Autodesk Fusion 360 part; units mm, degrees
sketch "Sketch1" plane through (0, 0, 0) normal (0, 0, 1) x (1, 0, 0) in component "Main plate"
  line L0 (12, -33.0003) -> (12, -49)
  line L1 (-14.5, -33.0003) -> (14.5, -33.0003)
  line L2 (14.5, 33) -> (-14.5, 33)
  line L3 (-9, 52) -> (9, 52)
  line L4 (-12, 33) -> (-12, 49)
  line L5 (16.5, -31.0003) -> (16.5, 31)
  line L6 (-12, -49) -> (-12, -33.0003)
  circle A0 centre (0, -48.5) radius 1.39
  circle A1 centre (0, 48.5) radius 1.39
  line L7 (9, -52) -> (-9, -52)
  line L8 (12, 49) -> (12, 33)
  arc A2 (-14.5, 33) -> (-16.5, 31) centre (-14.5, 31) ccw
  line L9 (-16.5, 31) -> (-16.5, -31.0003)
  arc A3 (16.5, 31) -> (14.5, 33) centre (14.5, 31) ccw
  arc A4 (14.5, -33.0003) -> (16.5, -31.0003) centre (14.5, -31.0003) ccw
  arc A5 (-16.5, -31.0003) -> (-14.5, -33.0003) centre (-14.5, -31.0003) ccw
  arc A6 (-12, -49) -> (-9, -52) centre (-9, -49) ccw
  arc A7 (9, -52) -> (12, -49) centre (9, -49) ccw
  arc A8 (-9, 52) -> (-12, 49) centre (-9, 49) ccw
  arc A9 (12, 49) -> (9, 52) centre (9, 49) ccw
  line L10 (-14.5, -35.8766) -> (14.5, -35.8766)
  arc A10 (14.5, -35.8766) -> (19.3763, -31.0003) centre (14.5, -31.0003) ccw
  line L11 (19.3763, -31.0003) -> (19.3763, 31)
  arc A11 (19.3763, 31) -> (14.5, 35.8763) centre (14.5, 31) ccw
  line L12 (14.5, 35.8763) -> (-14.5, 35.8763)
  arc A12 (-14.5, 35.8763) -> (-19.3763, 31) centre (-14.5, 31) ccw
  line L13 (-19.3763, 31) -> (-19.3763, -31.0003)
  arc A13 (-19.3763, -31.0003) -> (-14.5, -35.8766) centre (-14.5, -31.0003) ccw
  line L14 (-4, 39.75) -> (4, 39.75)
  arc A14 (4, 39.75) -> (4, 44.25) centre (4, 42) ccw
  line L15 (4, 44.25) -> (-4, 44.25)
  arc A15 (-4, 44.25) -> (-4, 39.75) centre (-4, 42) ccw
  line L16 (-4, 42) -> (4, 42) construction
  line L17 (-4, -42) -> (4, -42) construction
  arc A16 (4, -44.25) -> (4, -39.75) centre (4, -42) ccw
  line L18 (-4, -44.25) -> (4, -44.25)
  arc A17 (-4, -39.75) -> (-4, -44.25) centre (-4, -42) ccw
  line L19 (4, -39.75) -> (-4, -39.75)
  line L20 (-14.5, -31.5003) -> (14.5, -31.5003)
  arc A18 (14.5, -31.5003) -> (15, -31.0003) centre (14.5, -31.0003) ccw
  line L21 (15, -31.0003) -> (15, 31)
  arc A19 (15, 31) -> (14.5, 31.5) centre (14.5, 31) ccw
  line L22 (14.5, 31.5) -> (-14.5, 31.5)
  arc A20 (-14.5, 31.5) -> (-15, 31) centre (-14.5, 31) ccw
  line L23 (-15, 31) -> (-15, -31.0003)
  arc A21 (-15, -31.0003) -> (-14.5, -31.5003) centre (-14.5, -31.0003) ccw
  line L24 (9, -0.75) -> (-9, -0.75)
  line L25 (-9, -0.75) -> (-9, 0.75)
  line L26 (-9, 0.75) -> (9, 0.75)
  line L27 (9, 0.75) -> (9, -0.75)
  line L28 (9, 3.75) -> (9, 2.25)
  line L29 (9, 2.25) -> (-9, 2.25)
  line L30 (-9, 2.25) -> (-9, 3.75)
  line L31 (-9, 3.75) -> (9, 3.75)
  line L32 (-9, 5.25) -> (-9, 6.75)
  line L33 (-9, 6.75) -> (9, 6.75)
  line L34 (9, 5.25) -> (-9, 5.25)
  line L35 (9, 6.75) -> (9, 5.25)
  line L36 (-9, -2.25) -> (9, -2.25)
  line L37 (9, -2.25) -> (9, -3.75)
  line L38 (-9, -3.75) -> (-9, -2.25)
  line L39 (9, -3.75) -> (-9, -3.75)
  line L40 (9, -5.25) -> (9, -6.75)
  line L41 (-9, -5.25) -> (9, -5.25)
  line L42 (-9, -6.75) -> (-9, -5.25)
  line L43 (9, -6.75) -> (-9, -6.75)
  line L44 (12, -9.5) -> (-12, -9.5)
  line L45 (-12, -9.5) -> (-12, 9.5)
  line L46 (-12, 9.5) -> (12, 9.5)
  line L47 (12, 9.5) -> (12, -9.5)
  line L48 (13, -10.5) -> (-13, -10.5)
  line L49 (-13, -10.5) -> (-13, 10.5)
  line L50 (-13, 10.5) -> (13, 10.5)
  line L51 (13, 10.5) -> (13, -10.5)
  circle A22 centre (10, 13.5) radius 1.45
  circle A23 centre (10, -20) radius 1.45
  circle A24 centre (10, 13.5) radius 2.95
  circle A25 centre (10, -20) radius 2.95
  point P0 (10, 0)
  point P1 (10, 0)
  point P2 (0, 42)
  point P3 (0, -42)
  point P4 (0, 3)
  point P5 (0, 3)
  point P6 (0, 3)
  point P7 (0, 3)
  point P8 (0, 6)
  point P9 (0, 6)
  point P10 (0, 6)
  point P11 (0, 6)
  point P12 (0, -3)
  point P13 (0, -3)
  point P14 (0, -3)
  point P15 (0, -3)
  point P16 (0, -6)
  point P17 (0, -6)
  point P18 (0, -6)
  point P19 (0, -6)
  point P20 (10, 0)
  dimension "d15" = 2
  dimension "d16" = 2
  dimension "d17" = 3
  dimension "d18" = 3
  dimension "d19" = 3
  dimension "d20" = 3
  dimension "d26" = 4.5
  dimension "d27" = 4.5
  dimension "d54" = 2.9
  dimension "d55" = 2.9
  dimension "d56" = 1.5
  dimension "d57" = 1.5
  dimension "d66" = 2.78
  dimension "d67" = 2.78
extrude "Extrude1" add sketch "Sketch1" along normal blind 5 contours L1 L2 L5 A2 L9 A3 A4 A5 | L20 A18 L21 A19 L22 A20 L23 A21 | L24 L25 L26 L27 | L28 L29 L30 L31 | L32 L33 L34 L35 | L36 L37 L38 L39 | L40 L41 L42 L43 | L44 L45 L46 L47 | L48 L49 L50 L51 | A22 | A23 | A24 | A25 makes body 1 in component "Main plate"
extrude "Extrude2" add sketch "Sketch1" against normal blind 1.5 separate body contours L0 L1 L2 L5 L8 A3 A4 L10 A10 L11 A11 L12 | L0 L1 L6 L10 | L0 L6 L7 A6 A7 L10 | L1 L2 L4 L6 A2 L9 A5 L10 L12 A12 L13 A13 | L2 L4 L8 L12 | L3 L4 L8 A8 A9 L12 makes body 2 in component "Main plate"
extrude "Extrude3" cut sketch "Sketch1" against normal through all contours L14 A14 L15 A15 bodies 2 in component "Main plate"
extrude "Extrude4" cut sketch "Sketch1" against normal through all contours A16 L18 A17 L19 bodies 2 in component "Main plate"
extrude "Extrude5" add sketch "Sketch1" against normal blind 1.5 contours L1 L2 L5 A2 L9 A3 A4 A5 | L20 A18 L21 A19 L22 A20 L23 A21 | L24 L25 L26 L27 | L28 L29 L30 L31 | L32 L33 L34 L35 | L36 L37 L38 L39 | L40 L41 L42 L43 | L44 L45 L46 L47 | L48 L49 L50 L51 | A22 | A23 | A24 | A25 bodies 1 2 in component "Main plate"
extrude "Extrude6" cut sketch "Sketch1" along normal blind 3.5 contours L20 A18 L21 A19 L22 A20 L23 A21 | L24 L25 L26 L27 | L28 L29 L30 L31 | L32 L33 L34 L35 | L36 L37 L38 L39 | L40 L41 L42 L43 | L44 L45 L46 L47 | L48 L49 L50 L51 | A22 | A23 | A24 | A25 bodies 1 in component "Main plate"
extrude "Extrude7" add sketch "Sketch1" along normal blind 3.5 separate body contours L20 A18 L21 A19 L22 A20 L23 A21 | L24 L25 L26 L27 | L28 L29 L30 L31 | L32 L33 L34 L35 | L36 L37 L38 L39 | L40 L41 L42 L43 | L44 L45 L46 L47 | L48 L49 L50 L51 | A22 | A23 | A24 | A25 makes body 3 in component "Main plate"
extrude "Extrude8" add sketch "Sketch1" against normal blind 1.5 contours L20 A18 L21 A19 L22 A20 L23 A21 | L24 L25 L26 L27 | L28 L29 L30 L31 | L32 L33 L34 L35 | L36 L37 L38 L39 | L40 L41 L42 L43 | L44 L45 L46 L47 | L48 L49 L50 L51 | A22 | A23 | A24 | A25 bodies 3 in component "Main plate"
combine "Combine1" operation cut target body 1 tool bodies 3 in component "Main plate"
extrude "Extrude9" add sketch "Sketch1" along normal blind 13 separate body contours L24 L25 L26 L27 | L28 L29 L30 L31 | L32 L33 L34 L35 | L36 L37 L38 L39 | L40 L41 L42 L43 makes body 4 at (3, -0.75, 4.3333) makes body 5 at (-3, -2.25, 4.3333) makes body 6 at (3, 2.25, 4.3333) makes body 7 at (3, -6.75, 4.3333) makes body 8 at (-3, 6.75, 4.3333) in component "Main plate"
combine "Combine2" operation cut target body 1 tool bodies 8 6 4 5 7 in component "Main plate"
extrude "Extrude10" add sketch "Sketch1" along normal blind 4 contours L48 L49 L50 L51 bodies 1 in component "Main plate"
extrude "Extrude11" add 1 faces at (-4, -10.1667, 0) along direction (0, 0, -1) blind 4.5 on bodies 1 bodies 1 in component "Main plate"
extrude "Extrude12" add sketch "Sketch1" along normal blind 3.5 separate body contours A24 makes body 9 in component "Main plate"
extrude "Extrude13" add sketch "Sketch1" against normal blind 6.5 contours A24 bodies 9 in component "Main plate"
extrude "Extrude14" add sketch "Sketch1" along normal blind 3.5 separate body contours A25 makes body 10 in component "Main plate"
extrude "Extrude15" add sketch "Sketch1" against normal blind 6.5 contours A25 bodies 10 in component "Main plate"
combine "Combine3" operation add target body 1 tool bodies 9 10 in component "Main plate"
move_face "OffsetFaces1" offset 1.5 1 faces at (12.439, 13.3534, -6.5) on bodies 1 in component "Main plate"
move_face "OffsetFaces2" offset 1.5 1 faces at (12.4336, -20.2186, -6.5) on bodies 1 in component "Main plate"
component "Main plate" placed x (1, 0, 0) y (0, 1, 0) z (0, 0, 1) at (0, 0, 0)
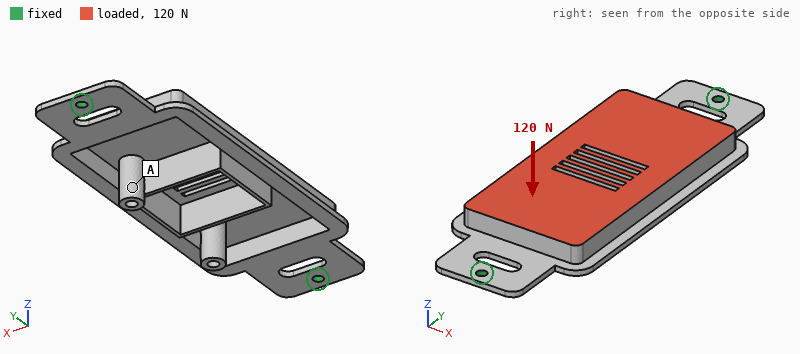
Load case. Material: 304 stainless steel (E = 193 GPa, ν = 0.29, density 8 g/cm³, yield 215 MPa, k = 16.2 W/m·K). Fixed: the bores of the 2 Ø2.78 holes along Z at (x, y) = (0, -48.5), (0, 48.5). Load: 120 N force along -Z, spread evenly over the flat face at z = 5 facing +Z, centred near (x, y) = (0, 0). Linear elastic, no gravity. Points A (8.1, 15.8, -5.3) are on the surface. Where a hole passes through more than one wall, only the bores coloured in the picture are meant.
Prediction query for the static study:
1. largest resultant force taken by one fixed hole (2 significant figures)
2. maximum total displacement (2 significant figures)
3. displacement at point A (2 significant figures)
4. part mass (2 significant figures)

150 N
51 µm
48 µm
60 g
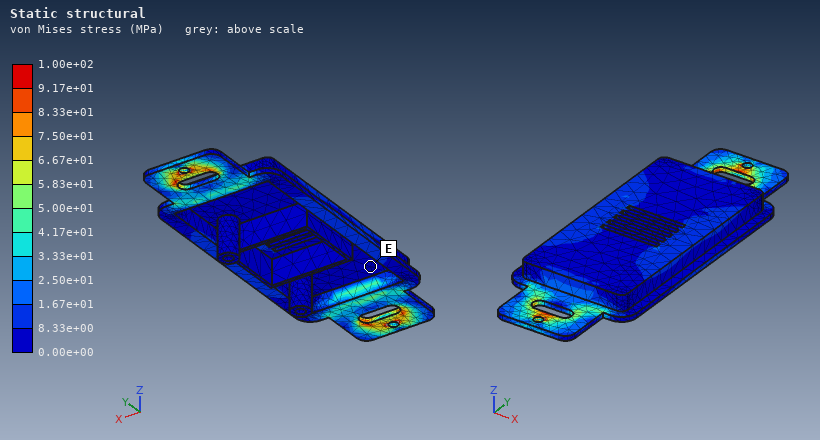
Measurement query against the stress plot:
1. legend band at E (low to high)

0.00e+00 to 8.33e+00 MPa
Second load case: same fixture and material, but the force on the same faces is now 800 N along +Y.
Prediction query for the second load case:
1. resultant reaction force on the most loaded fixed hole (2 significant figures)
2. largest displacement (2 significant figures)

400 N
21 µm
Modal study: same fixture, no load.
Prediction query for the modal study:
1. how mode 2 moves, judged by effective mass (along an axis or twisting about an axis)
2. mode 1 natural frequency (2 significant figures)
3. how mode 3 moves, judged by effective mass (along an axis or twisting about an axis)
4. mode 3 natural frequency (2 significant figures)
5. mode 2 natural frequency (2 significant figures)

along Z
820 Hz
twisting about X
2200 Hz
1100 Hz
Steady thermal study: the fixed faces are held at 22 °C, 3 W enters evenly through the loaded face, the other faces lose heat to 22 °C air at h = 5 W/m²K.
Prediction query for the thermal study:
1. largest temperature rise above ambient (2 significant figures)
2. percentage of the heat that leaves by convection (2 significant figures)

48 K
60 %
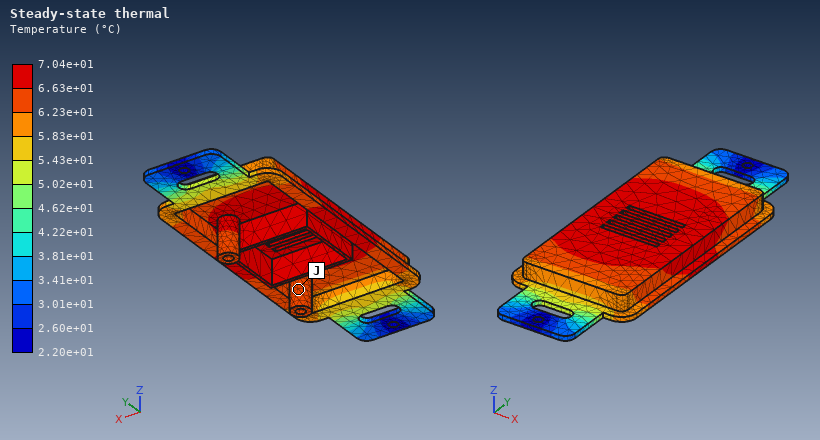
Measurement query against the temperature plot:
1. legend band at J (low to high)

6.23e+01 to 6.63e+01 °C
